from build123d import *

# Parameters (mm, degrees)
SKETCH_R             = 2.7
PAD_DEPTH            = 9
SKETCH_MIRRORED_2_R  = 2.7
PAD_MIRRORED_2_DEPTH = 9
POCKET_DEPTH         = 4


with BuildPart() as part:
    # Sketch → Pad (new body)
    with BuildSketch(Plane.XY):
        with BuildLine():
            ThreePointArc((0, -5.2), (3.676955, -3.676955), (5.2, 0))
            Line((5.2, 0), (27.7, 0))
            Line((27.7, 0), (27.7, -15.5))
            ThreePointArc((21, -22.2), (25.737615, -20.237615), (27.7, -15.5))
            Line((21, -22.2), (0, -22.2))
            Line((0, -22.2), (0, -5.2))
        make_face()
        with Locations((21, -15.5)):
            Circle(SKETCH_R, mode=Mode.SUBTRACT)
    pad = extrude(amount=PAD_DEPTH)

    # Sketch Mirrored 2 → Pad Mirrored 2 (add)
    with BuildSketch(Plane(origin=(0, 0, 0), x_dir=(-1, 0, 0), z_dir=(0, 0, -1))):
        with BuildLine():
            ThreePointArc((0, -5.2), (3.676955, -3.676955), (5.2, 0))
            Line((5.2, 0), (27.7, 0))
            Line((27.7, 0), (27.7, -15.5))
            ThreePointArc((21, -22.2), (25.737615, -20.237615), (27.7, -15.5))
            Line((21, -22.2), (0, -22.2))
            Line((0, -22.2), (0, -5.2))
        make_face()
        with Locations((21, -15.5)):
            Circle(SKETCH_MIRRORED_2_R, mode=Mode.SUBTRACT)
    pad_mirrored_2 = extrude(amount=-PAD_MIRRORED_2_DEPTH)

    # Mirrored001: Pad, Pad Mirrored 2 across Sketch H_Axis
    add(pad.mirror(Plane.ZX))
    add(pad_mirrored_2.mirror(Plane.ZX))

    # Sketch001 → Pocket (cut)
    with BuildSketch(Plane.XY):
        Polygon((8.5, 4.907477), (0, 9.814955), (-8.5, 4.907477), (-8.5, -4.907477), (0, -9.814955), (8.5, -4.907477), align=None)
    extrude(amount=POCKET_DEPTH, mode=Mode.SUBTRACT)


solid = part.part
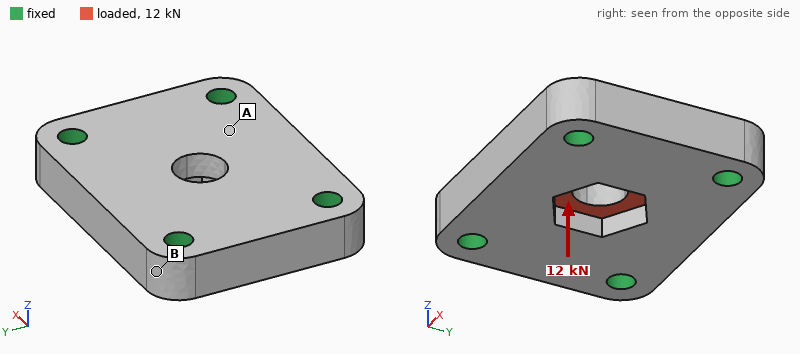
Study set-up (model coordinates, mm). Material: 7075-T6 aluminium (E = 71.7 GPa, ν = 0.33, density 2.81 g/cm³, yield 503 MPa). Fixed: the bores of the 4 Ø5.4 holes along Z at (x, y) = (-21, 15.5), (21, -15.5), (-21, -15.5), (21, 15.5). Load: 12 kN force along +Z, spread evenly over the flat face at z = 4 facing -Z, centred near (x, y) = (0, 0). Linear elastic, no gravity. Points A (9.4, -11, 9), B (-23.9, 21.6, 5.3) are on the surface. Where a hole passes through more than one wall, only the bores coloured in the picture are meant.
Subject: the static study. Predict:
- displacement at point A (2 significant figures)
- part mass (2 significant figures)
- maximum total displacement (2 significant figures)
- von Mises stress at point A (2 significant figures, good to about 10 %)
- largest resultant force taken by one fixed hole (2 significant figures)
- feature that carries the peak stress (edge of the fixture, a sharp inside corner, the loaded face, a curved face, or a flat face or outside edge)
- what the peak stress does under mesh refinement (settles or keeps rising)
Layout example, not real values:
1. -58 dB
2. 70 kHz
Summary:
1. 33 µm
2. 55 g
3. 78 µm
4. 61 MPa
5. 3.1 kN
6. edge of the fixture
7. keeps rising
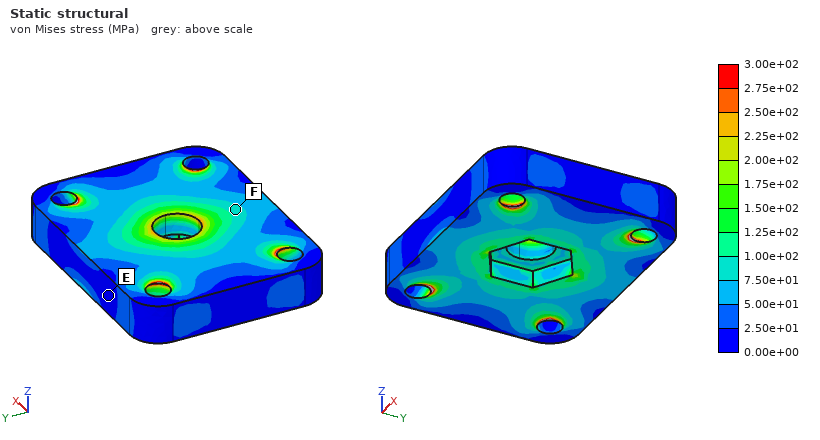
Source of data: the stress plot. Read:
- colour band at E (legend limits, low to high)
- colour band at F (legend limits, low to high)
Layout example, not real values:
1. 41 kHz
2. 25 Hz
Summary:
1. 0.00e+00 to 2.50e+01 MPa
2. 7.50e+01 to 1.00e+02 MPa
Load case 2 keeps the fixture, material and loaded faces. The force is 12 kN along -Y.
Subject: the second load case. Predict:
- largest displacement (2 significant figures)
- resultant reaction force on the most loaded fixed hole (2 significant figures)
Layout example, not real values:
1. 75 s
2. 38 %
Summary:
1. 22 µm
2. 3.4 kN
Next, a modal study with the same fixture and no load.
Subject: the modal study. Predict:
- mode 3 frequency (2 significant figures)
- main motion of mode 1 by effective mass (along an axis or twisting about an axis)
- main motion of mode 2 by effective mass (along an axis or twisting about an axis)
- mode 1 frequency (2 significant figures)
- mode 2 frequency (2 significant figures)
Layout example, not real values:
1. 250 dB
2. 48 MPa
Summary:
1. 31 kHz
2. along Z
3. twisting about X
4. 20 kHz
5. 25 kHz
